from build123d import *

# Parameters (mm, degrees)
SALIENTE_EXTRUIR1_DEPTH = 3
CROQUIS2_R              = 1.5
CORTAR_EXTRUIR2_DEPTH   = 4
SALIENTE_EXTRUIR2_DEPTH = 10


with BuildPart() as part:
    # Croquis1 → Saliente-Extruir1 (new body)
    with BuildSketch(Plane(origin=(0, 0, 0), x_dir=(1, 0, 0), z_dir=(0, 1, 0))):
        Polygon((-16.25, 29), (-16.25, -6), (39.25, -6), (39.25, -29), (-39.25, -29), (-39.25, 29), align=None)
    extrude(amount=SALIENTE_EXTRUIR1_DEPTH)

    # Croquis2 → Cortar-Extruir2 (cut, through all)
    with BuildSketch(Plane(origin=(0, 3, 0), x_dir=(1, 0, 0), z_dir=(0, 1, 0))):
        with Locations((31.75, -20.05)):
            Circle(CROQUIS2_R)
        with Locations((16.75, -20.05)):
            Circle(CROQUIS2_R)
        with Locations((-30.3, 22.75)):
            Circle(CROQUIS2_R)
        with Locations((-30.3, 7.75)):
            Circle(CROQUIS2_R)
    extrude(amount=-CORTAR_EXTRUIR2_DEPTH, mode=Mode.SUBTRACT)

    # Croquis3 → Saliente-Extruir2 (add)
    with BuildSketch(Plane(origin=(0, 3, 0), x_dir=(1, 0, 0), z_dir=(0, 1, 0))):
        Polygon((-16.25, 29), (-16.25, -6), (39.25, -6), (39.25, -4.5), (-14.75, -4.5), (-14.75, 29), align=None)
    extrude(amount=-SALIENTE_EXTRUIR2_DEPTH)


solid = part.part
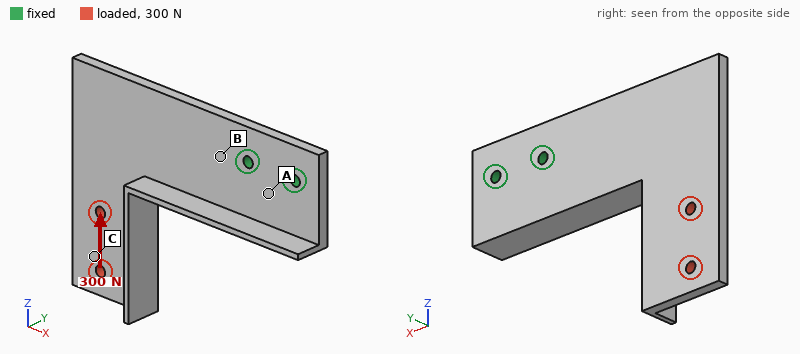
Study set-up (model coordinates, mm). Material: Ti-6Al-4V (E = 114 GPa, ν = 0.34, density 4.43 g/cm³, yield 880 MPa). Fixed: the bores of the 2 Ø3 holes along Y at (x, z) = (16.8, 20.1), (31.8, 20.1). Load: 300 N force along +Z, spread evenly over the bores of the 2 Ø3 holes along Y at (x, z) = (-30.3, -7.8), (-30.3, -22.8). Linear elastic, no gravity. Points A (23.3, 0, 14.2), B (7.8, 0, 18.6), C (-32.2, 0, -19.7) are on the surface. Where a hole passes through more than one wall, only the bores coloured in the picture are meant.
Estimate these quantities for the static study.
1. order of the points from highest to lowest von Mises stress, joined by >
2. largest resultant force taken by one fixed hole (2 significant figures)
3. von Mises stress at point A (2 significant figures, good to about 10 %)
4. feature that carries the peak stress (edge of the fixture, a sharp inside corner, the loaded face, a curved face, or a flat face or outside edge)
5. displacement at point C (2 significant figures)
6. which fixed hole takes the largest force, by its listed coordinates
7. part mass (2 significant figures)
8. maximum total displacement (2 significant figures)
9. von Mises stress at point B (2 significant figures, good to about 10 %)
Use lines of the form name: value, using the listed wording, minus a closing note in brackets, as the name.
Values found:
order of the points from highest to lowest von Mises stress, joined by >: A > B > C
largest resultant force taken by one fixed hole: 1.1 kN
von Mises stress at point A: 29 MPa
feature that carries the peak stress: edge of the fixture
displacement at point C: 0.084 mm
which fixed hole takes the largest force, by its listed coordinates: (16.8, 20.1)
part mass: 40 g
maximum total displacement: 0.10 mm
von Mises stress at point B: 16 MPa
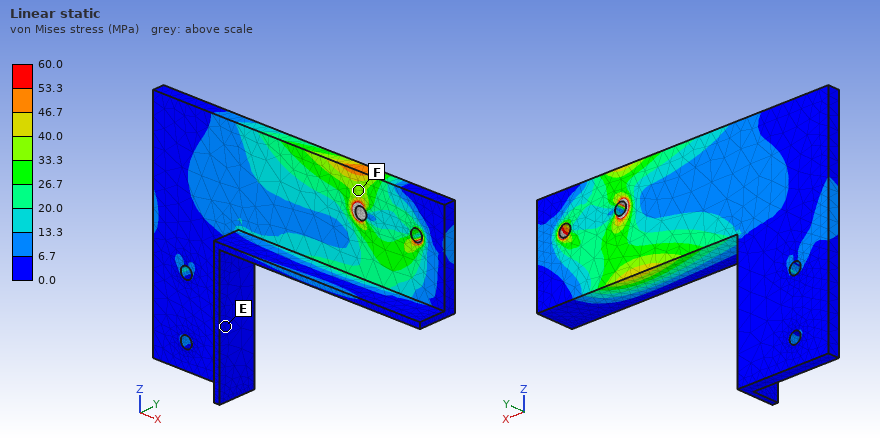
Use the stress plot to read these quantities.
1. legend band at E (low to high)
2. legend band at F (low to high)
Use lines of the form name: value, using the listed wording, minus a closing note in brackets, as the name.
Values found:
legend band at E: 0.0 to 6.7 MPa
legend band at F: 33.3 to 40.0 MPa
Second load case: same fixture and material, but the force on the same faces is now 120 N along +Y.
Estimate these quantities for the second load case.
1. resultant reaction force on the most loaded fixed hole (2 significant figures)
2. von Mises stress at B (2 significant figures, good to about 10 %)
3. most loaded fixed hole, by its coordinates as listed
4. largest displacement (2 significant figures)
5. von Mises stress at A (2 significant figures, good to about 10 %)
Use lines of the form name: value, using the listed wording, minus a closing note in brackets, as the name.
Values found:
resultant reaction force on the most loaded fixed hole: 360 N
von Mises stress at B: 100 MPa
most loaded fixed hole, by its coordinates as listed: (16.8, 20.1)
largest displacement: 1.2 mm
von Mises stress at A: 76 MPa
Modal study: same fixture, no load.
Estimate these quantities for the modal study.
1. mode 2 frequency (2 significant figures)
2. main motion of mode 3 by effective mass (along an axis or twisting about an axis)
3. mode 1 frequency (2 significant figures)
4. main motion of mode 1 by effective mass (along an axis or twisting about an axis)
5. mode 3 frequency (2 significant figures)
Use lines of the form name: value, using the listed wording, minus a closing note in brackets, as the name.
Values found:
mode 2 frequency: 1200 Hz
main motion of mode 3 by effective mass: along Z
mode 1 frequency: 580 Hz
main motion of mode 1 by effective mass: along Y
mode 3 frequency: 2400 Hz
